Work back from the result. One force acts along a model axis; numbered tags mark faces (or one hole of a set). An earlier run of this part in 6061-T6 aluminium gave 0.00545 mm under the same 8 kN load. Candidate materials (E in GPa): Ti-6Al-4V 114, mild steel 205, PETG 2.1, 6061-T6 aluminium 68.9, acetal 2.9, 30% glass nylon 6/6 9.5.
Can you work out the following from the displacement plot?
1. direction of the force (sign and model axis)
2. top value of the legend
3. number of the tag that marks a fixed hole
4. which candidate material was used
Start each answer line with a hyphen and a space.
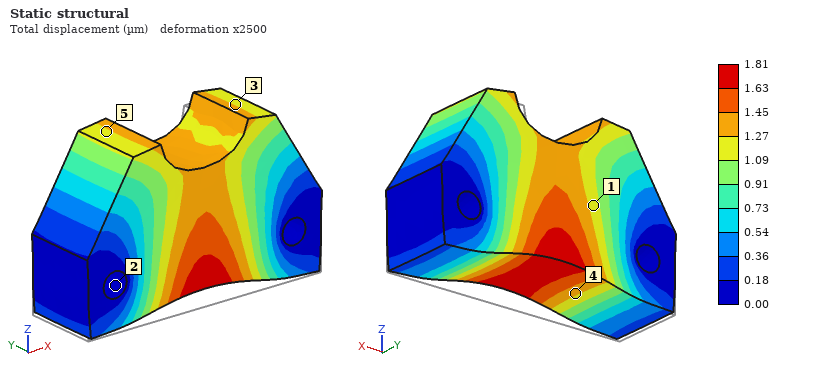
- +Z
- 1.81 µm
- 2
- mild steel
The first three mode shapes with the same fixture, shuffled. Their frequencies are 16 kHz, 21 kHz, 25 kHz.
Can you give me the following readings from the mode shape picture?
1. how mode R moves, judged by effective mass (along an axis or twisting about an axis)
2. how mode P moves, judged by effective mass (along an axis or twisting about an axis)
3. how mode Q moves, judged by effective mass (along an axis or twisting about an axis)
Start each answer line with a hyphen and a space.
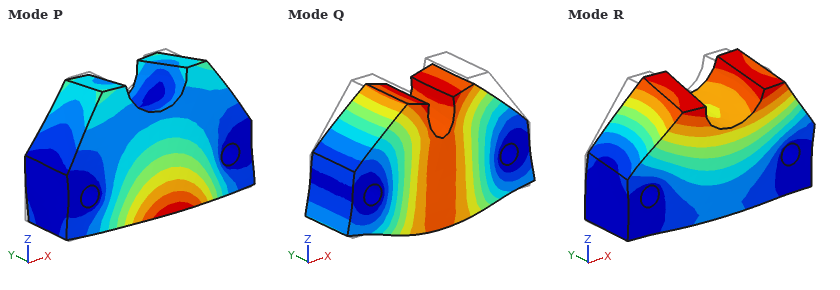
- along Y
- along Y
- along Z
